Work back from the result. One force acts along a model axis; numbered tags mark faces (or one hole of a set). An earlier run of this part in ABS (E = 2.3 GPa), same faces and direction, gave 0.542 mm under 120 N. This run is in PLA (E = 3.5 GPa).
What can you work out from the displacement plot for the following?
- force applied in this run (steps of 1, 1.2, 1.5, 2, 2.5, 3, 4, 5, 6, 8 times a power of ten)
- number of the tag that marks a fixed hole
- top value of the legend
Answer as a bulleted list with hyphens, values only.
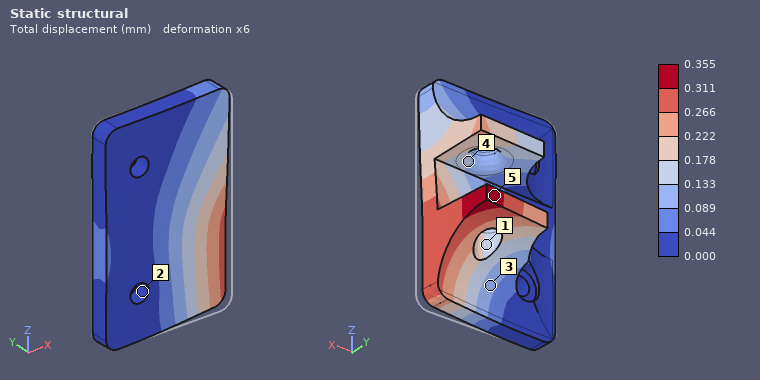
- 120 N
- 2
- 0.355 mm
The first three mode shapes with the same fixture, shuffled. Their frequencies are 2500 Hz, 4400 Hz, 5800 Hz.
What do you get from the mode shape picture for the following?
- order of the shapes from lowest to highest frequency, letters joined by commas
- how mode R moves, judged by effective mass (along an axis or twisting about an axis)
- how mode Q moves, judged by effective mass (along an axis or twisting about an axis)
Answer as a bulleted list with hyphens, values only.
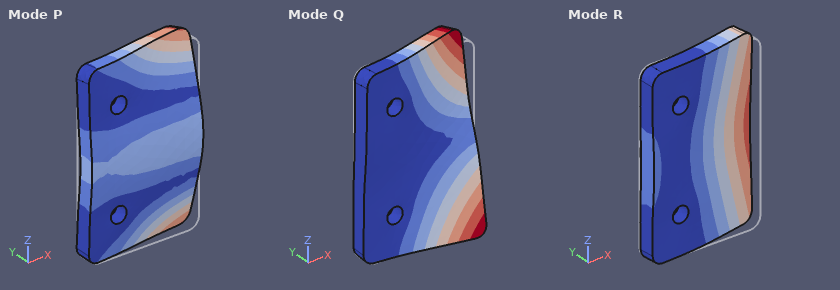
- R, Q, P
- along Y
- twisting about X
